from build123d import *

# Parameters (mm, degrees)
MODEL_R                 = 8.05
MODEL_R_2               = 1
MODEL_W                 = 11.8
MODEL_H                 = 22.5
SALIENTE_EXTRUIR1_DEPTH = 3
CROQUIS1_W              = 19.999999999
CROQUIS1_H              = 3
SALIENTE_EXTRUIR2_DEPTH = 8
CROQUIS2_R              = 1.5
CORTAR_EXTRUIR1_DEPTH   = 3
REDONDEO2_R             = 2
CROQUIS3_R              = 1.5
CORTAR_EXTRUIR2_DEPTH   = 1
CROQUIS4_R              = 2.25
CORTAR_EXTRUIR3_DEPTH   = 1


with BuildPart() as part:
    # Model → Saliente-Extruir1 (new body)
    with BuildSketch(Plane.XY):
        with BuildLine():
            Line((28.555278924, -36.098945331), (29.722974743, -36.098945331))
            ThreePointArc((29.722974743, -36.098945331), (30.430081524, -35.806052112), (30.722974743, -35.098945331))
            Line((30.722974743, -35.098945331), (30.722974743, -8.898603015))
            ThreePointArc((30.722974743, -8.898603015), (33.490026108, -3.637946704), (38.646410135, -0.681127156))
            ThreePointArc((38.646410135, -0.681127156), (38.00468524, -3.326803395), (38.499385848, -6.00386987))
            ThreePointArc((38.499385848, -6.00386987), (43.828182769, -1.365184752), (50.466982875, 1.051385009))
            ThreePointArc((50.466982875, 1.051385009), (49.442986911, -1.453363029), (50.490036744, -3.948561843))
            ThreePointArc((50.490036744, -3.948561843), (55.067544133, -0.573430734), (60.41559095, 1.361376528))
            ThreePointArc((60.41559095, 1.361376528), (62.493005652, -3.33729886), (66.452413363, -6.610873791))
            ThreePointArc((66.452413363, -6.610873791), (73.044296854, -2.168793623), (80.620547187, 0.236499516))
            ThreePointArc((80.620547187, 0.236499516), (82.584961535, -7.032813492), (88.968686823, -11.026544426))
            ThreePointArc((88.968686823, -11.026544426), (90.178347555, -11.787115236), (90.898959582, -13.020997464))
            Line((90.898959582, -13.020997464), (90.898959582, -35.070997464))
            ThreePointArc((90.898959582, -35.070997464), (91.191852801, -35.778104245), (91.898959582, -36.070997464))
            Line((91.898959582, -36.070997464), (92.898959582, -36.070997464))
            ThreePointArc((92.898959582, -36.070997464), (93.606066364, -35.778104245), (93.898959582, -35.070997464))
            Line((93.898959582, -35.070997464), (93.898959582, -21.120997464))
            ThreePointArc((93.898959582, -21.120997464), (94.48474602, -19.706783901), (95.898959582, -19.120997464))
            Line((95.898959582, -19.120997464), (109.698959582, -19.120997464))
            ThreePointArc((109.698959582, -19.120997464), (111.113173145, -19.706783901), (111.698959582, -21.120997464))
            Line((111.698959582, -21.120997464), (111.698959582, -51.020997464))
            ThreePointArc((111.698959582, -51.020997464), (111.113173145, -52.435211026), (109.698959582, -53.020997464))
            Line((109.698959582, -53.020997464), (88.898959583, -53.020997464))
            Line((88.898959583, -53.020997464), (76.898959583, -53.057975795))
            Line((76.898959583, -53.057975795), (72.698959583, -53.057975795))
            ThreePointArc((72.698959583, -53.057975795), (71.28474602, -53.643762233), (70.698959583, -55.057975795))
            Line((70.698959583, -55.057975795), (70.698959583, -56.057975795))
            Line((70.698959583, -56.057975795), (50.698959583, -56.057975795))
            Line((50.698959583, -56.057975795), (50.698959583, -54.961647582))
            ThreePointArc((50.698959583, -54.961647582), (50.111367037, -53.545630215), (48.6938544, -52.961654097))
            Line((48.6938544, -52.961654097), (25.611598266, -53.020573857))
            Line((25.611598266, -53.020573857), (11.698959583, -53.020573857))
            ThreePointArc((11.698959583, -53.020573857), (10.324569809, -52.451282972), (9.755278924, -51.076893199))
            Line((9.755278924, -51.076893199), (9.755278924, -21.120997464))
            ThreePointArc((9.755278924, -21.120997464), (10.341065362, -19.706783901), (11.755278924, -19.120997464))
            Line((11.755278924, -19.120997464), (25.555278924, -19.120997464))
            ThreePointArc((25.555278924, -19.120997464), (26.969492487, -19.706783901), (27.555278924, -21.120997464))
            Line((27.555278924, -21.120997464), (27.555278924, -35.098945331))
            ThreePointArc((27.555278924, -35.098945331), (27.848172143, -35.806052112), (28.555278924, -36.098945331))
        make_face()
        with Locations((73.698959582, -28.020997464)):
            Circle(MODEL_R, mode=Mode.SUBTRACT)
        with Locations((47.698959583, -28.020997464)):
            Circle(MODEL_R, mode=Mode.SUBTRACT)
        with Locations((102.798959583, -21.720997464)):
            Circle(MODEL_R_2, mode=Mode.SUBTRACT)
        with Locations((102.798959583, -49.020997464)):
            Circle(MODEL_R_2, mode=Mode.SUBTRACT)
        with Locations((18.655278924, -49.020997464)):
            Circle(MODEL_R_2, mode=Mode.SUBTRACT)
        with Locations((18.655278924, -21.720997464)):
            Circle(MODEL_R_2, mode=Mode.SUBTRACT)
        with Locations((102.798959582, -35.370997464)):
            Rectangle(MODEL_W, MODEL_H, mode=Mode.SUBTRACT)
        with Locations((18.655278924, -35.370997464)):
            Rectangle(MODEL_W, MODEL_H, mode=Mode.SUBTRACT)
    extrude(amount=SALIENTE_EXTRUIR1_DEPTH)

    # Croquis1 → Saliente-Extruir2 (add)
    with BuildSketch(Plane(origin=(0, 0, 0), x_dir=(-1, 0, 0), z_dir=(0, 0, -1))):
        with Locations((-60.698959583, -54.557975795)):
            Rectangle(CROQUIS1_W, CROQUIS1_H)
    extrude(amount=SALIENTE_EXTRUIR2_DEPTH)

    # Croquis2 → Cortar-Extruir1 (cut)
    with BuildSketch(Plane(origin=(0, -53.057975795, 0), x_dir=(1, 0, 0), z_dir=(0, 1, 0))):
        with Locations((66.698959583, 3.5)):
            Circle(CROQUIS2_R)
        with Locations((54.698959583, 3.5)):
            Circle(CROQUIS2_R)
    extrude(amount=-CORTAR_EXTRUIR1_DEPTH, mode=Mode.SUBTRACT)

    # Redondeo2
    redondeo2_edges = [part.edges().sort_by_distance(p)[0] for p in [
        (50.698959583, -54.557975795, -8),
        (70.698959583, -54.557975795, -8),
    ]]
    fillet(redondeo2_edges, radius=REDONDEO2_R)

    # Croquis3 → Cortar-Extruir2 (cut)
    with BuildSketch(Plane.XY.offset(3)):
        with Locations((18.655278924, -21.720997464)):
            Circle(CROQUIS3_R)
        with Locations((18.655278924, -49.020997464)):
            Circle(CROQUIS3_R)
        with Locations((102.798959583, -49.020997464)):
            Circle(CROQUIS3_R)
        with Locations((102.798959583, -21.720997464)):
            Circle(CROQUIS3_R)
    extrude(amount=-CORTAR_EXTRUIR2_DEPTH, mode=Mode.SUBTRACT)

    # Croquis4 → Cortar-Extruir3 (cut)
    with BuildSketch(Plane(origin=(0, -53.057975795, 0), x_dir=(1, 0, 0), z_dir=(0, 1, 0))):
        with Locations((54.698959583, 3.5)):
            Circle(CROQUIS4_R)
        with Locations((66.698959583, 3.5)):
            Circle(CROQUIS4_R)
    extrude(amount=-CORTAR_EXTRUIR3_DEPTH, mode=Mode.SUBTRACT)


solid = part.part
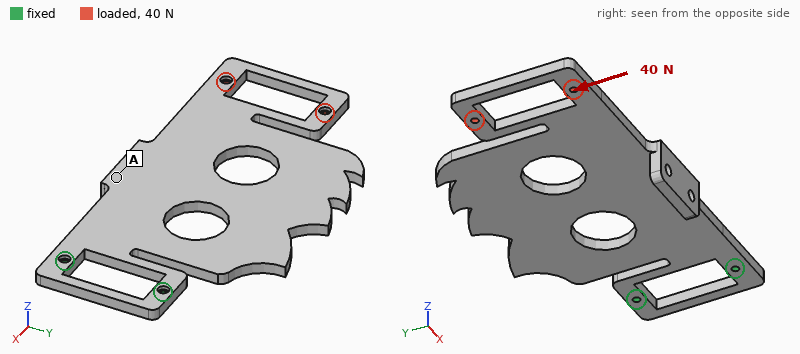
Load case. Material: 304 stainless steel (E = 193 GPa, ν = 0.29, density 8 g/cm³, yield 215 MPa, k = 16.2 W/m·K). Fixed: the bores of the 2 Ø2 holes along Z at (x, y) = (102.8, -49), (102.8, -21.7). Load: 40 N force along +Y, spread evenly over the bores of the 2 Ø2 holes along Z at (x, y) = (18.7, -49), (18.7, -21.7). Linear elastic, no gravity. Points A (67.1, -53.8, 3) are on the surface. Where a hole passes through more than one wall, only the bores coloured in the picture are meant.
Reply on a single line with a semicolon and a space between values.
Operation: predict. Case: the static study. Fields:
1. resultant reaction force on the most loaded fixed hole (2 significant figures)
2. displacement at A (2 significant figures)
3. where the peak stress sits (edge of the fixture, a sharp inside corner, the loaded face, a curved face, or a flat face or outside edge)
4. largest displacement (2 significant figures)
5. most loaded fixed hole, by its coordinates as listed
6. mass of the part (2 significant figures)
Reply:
150 N; 0.032 mm; a curved face; 0.10 mm; (102.8, -21.7); 85 g
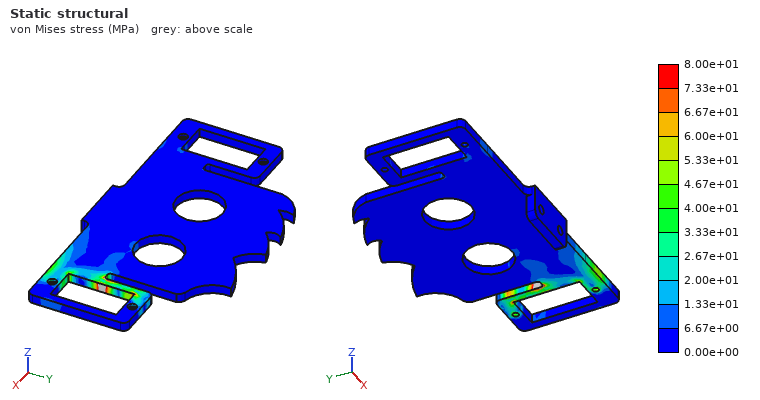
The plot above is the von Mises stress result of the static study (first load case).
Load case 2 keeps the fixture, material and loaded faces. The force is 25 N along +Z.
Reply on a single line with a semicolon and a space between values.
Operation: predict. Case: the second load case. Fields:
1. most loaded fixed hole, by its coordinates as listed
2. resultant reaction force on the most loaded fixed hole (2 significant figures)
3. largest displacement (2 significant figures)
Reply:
(102.8, -21.7); 16 N; 1.0 mm
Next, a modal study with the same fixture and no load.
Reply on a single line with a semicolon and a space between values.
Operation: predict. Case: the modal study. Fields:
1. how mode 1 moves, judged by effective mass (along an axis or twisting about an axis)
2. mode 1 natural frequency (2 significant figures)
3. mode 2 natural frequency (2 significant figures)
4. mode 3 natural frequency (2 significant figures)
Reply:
along Z; 170 Hz; 590 Hz; 610 Hz
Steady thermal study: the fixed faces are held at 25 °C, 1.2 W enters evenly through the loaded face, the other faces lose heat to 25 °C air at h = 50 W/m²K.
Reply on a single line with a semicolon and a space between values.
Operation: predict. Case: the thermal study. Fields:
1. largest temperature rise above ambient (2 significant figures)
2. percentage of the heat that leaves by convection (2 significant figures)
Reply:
26 K; 100 %
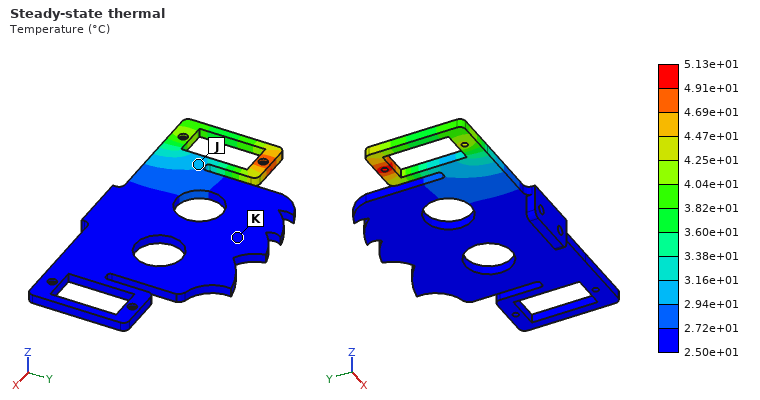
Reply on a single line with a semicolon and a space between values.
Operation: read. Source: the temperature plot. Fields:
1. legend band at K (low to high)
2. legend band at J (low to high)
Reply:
2.50e+01 to 2.72e+01 °C; 2.94e+01 to 3.16e+01 °C
